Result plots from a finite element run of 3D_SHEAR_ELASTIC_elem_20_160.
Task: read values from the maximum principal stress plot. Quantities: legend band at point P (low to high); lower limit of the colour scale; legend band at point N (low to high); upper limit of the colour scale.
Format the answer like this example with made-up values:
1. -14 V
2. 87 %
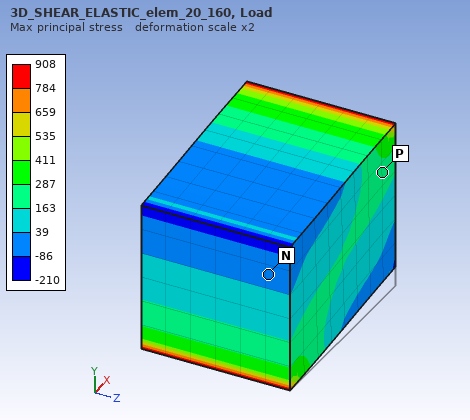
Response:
1. 163 to 287
2. -210
3. -86 to 39
4. 908
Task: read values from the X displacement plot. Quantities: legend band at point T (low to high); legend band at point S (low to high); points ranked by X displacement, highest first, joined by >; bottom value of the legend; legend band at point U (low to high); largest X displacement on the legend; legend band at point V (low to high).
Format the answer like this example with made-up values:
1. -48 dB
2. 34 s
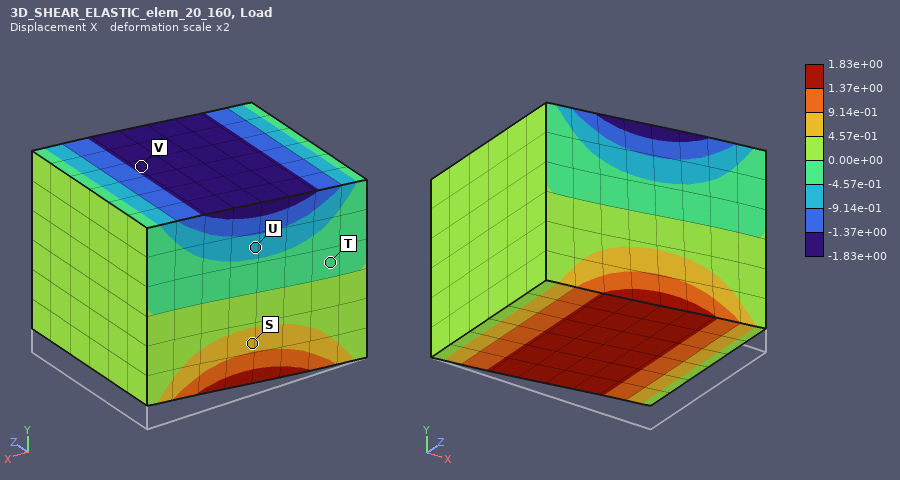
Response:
1. -4.57e-01 to 0.00e+00
2. 4.57e-01 to 9.14e-01
3. S > T > U > V
4. -1.83e+00
5. -9.14e-01 to -4.57e-01
6. 1.83e+00
7. -1.83e+00 to -1.37e+00
